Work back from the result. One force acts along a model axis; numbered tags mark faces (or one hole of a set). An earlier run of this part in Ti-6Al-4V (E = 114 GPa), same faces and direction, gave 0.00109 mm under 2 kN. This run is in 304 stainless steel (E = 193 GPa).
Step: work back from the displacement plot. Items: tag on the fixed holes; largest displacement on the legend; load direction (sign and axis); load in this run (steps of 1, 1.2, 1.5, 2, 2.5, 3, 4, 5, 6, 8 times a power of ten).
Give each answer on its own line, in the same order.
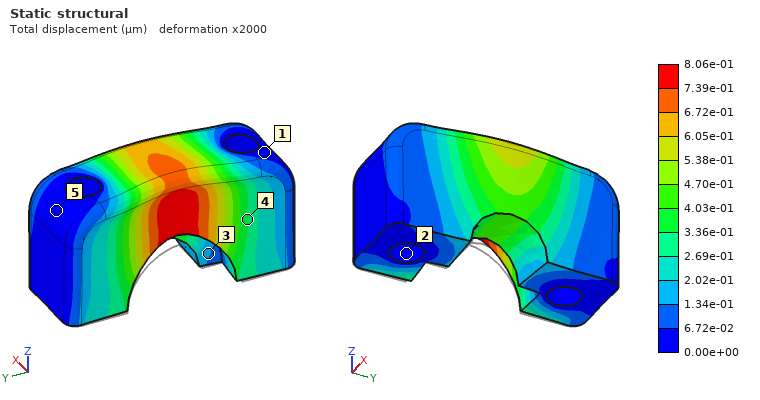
2
8.06e-01 µm
+X
2.5 kN
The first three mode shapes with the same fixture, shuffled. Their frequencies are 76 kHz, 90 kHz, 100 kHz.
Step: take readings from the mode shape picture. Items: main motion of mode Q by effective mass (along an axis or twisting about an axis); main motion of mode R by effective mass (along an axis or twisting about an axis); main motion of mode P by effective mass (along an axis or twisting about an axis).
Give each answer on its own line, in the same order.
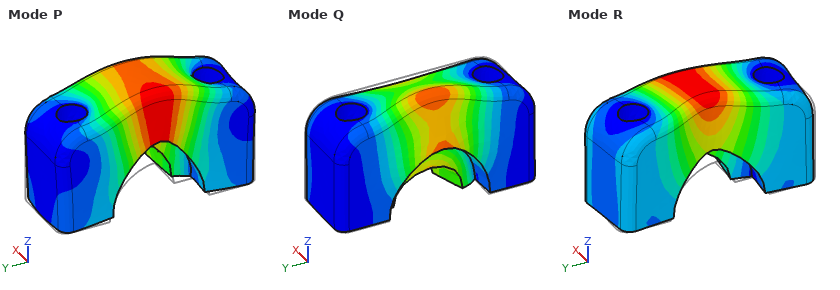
twisting about Y
along X
along Z
